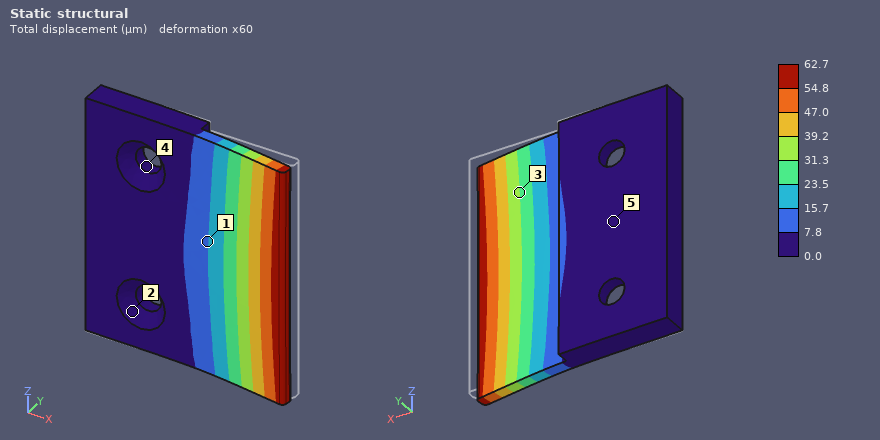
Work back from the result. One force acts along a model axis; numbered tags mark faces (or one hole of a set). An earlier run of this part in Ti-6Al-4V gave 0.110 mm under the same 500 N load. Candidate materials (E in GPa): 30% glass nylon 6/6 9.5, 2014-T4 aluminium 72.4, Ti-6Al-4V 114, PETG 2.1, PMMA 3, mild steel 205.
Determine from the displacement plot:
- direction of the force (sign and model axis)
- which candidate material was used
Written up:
-Y
mild steel
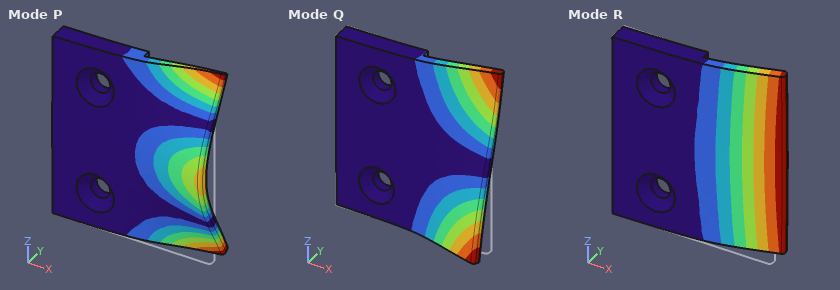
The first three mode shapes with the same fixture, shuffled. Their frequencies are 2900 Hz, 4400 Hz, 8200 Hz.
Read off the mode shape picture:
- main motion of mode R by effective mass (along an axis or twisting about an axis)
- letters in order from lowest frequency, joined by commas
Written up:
along Y
R, Q, P
